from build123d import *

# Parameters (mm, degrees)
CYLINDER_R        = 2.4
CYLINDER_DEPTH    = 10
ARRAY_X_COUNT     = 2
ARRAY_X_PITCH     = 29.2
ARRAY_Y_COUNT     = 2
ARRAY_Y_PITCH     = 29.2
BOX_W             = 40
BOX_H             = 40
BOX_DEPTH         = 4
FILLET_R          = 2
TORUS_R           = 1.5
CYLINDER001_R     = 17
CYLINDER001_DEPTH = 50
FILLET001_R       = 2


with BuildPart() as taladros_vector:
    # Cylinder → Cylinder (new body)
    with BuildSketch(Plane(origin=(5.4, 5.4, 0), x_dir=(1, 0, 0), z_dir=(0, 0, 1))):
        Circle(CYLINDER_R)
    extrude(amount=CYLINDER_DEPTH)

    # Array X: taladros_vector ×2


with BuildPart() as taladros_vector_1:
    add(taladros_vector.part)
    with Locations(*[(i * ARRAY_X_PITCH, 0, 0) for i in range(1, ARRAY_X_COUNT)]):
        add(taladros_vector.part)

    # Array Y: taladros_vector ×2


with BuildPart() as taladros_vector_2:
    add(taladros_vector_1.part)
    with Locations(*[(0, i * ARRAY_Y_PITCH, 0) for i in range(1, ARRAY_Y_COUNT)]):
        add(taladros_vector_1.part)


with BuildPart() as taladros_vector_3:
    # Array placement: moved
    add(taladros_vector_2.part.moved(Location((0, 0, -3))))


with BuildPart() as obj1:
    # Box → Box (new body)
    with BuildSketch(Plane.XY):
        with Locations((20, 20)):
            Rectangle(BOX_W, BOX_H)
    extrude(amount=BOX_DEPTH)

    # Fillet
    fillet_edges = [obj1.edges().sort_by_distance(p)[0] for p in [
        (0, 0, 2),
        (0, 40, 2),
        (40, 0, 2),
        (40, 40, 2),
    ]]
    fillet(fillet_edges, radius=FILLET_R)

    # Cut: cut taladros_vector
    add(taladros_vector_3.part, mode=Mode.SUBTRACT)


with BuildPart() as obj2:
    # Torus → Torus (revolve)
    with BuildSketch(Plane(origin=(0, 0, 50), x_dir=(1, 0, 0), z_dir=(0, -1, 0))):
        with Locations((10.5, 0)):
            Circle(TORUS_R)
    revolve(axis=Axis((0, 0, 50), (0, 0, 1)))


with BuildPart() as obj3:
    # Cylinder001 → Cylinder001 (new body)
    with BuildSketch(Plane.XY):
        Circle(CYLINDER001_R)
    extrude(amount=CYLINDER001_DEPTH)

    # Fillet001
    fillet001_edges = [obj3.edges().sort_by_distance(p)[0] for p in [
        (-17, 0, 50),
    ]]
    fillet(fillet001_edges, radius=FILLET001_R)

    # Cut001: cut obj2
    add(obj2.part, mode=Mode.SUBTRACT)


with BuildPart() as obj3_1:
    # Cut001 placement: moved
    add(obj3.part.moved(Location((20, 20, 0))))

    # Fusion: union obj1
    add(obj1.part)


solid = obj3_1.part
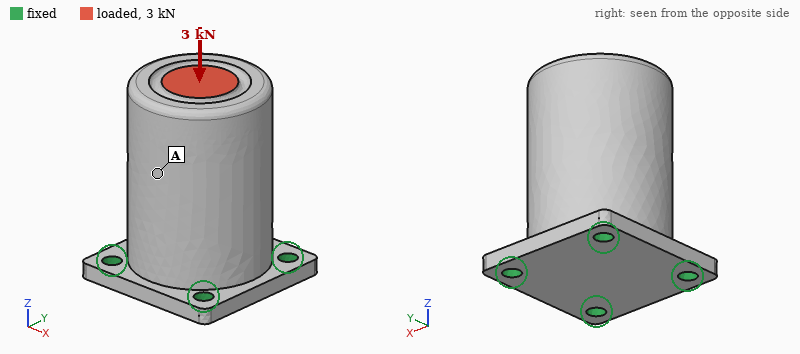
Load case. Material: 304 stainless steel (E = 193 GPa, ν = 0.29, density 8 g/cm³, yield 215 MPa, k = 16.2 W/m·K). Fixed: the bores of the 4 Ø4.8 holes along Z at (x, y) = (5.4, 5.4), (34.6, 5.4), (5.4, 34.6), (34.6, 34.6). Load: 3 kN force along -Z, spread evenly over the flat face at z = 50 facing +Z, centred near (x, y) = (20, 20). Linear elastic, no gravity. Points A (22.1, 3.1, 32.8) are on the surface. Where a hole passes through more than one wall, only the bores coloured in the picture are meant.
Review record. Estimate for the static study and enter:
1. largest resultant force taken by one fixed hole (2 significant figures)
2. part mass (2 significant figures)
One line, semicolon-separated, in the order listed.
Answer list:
810 N; 380 g
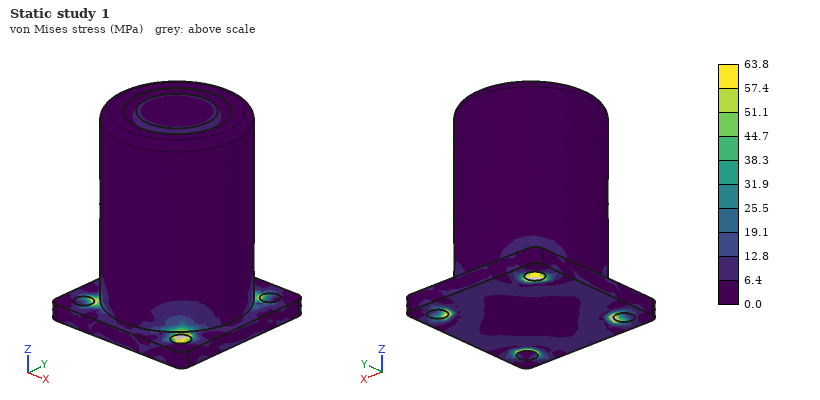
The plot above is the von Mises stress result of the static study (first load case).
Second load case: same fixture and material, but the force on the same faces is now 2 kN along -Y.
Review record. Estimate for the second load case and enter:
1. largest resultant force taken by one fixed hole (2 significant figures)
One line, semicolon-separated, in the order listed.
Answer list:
2.0 kN
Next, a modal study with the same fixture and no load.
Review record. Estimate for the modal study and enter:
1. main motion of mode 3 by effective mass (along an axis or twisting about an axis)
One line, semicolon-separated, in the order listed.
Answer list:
along Z
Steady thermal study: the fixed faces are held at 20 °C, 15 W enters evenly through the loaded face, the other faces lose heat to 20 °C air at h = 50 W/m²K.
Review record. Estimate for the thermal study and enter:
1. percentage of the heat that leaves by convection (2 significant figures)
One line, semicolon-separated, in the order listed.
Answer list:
54 %
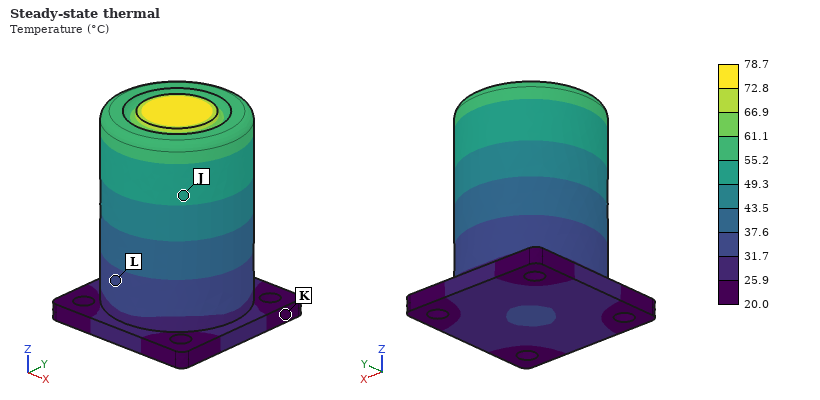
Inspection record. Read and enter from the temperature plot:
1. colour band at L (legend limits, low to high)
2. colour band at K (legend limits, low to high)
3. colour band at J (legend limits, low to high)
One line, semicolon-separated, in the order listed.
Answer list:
31.7 to 37.6 °C; 20.0 to 25.9 °C; 49.3 to 55.2 °C
